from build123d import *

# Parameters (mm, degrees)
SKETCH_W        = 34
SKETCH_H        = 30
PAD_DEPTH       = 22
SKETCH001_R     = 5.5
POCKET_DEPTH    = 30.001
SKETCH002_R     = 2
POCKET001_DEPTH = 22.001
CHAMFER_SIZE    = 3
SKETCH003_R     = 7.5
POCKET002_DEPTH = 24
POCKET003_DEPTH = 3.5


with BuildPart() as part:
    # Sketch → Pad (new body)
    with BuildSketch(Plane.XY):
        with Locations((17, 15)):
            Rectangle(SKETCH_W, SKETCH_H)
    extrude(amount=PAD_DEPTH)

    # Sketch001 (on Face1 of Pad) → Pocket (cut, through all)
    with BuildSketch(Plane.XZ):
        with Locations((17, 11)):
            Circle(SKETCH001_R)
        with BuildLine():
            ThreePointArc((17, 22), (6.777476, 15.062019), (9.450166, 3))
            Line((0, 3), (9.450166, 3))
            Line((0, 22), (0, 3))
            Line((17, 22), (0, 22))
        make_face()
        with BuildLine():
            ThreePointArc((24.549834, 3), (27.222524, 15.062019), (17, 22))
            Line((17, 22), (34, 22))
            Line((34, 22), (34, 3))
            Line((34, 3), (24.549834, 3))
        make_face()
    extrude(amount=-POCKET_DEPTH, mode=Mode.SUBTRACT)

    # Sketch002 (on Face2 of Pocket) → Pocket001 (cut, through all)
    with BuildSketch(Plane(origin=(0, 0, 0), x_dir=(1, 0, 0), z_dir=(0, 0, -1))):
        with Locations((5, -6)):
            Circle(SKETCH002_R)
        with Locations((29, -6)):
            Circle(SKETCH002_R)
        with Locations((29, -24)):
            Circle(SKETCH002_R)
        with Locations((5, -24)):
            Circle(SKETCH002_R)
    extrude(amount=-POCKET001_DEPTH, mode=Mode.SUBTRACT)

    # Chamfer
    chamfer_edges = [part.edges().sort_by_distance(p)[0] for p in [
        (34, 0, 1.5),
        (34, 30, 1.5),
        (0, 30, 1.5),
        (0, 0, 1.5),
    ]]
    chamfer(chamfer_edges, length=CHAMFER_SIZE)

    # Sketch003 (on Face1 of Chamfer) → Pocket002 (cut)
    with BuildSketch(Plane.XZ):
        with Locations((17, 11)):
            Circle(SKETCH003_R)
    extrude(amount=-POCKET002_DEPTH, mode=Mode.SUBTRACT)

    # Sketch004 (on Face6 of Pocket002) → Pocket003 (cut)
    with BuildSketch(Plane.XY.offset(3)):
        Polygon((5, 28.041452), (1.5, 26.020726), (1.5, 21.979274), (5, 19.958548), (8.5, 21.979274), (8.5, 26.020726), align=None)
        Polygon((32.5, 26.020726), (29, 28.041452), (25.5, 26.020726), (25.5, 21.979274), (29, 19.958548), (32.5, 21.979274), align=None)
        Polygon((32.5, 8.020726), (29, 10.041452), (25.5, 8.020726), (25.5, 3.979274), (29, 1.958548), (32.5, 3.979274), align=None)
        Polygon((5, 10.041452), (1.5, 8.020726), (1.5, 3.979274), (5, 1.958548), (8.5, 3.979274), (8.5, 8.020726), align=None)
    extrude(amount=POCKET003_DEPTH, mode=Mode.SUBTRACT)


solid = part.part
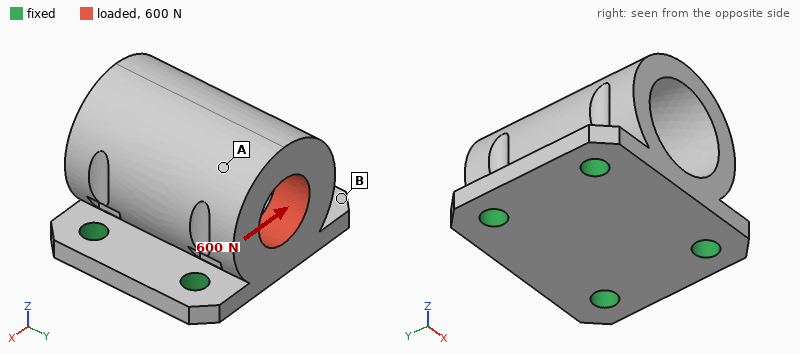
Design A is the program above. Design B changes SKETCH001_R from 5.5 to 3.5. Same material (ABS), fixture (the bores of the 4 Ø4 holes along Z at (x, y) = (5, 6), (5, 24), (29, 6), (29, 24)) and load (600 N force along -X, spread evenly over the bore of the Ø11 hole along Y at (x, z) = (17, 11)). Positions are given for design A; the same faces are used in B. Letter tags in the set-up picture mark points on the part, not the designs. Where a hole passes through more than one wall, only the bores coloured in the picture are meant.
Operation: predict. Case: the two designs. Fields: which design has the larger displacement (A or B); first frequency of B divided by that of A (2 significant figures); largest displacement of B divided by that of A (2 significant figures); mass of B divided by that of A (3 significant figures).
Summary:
A
1.0
0.77
1.04
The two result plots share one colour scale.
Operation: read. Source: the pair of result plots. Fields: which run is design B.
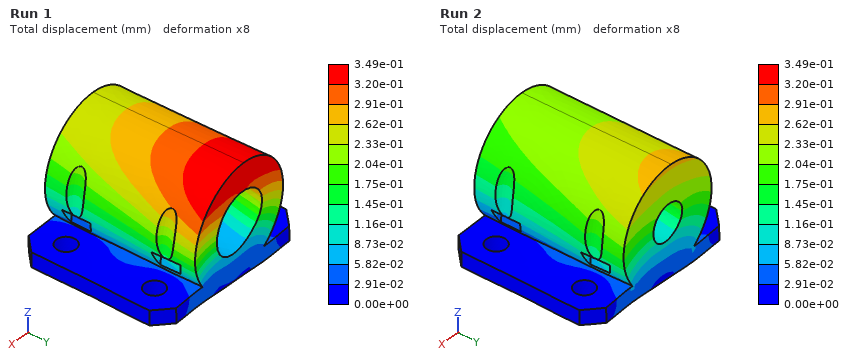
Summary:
Run 2
